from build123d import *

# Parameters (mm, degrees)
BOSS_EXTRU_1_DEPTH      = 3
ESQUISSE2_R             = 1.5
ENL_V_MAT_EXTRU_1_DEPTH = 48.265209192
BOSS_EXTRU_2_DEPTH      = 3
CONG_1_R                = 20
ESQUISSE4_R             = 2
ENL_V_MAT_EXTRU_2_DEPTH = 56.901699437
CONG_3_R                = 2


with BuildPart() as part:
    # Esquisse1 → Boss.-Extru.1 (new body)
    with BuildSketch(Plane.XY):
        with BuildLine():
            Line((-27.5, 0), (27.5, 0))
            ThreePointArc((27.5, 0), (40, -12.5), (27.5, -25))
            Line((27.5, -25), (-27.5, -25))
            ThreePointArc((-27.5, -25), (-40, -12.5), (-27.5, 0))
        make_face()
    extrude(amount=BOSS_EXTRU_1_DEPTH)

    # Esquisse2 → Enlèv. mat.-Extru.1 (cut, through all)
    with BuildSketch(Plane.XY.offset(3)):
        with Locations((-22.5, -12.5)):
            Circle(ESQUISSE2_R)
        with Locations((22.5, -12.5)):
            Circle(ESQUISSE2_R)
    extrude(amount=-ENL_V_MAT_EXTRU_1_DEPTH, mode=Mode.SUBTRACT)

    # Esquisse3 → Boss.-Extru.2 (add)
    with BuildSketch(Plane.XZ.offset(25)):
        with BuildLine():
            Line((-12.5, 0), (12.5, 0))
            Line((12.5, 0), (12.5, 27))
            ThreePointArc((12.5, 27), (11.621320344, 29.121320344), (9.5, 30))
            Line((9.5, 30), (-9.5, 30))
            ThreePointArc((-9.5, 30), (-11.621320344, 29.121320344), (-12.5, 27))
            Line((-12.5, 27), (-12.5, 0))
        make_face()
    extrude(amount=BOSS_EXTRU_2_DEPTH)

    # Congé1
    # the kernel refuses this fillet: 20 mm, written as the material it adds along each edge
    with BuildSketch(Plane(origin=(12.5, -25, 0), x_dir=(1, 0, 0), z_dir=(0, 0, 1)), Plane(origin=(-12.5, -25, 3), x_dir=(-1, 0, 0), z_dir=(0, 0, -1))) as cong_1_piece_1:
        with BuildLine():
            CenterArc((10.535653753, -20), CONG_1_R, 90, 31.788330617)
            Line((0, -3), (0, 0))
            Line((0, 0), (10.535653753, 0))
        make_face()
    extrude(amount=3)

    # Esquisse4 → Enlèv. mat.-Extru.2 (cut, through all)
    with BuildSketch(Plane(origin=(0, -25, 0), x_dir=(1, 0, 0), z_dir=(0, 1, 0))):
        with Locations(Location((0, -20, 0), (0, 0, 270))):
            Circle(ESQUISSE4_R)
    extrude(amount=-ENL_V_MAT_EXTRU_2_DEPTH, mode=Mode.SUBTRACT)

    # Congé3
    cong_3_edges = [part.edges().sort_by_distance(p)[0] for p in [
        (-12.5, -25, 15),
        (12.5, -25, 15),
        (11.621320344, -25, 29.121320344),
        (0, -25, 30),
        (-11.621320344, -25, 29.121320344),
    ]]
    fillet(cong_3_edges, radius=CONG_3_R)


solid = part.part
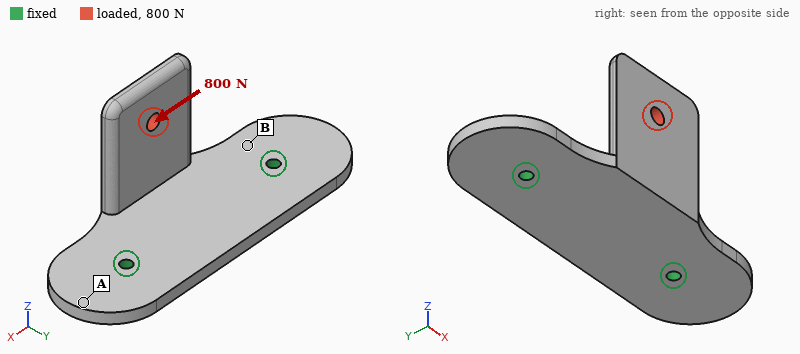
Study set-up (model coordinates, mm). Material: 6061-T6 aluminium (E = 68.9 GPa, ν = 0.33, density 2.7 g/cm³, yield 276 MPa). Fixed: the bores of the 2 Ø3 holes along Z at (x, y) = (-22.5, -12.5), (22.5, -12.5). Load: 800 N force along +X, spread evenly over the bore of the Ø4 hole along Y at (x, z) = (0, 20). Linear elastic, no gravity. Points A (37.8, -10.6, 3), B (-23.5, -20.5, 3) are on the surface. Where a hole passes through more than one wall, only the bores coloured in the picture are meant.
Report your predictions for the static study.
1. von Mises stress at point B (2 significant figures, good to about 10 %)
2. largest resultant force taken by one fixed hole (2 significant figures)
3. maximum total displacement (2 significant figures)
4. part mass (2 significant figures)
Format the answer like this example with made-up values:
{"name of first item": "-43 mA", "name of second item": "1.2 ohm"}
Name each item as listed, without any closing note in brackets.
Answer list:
{"von Mises stress at point B": "56 MPa", "largest resultant force taken by one fixed hole": "620 N", "maximum total displacement": "0.31 mm", "part mass": "21 g"}
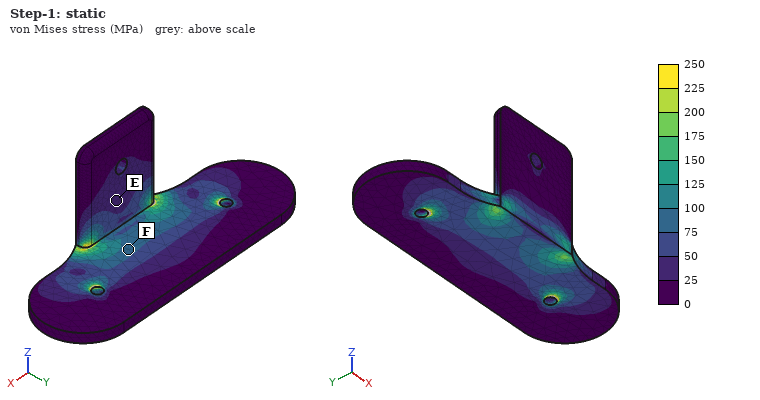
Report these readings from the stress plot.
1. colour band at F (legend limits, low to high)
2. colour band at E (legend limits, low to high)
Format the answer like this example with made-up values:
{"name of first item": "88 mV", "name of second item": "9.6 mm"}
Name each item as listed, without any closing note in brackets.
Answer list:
{"colour band at F": "75 to 100 MPa", "colour band at E": "25 to 50 MPa"}
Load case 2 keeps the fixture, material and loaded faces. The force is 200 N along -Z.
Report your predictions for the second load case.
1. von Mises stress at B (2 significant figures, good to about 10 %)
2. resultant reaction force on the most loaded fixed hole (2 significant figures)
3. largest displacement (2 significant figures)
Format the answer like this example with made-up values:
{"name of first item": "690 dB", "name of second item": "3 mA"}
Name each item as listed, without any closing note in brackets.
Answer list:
{"von Mises stress at B": "27 MPa", "resultant reaction force on the most loaded fixed hole": "100 N", "largest displacement": "0.13 mm"}
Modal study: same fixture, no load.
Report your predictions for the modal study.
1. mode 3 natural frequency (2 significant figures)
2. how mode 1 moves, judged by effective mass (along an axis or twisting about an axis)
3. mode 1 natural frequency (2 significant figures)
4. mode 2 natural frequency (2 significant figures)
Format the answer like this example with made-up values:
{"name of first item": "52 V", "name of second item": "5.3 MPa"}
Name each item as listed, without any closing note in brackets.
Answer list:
{"mode 3 natural frequency": "4500 Hz", "how mode 1 moves, judged by effective mass": "along Y", "mode 1 natural frequency": "1900 Hz", "mode 2 natural frequency": "4400 Hz"}
